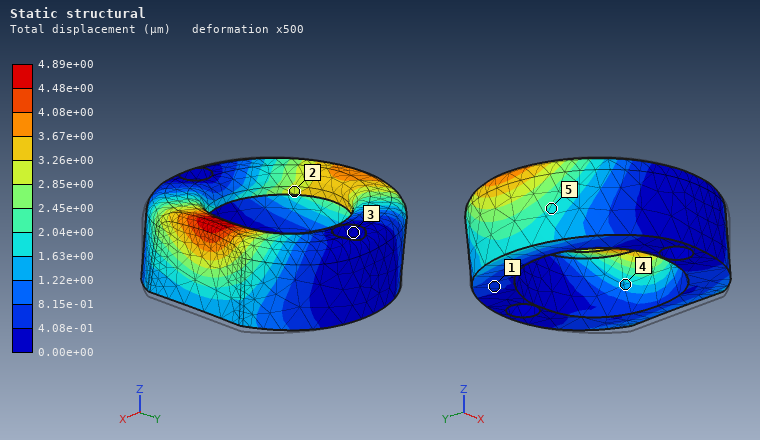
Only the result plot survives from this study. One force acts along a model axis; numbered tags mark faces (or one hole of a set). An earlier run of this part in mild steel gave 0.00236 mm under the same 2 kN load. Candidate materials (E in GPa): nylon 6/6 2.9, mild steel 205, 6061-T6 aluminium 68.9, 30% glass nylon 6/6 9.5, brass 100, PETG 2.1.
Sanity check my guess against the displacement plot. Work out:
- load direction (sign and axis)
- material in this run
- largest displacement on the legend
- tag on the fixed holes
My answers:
-X
brass
4.89e+00 µm
3
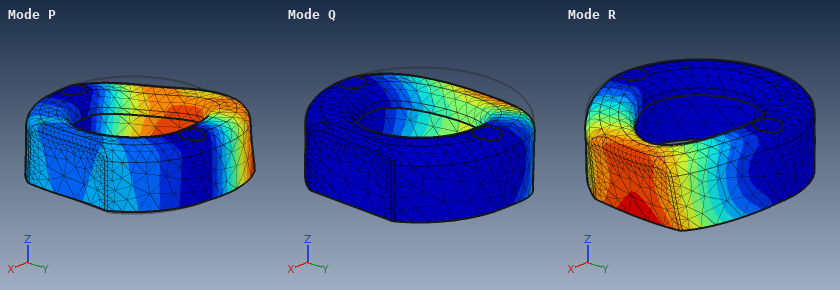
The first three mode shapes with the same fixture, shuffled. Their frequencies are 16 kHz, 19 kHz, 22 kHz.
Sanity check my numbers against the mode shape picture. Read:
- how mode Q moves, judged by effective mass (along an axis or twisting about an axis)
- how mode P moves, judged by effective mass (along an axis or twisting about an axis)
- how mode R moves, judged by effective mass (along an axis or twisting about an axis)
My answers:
along Z
along Y
along Z
